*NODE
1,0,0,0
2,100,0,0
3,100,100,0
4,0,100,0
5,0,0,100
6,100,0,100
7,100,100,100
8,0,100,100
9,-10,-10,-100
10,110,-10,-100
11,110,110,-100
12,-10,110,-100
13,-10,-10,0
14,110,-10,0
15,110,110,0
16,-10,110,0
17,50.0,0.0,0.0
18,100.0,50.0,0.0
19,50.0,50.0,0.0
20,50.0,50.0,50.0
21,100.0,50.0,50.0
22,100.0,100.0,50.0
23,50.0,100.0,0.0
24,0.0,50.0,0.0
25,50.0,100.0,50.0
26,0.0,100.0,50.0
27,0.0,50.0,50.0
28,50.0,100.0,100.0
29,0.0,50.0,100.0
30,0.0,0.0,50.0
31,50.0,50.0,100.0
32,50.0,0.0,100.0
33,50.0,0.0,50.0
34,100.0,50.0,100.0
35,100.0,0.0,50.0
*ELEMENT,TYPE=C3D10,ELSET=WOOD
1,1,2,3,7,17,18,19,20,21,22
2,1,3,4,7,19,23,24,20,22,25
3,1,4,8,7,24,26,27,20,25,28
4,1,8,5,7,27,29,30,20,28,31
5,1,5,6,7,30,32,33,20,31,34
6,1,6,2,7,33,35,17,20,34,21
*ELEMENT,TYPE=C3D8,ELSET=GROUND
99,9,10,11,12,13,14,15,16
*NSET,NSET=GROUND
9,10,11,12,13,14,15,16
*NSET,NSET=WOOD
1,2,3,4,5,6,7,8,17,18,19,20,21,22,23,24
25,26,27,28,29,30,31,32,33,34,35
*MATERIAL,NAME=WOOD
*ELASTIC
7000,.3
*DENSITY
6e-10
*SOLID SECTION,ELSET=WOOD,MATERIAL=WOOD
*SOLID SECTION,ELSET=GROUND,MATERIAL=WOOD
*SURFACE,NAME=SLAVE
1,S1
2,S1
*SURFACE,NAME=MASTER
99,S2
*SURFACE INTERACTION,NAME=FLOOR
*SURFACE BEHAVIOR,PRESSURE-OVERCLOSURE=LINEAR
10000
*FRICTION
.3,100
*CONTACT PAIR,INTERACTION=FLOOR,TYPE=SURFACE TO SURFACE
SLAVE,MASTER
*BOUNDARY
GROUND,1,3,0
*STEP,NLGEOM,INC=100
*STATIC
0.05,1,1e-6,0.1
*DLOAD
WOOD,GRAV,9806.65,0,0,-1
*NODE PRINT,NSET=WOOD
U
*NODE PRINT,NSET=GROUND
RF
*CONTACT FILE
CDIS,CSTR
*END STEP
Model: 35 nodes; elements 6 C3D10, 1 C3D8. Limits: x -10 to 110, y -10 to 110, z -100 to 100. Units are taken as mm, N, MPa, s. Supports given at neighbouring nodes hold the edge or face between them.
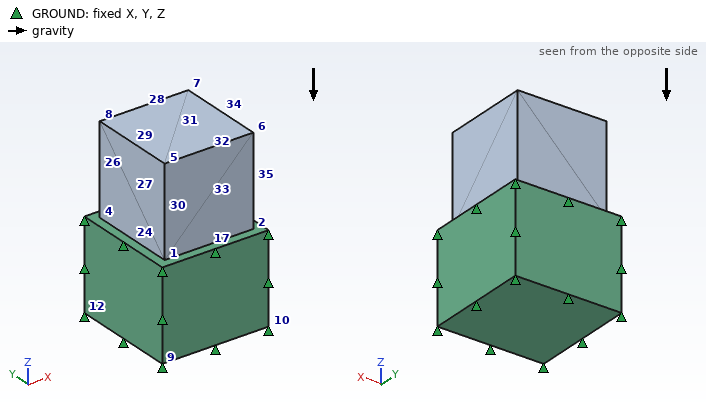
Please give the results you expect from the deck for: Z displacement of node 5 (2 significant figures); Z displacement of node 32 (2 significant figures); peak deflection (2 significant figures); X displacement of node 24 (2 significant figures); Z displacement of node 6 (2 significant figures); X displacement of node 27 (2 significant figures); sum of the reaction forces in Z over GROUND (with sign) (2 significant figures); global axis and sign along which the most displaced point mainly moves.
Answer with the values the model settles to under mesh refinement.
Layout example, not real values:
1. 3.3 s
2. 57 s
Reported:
1. -4.0e-06 mm
2. -4.1e-06 mm
3. 4.3e-06 mm
4. -8.6e-07 mm
5. -3.7e-06 mm
6. -6.7e-07 mm
7. 5.9 N
8. -Z
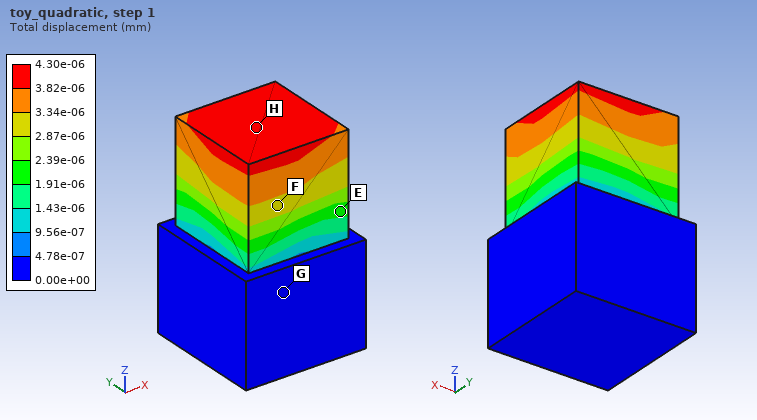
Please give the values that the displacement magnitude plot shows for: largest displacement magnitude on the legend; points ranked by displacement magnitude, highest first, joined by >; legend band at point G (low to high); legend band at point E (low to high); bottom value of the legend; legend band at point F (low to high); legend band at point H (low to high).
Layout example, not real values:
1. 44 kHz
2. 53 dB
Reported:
1. 4.30e-06 mm
2. H > F > E > G
3. 0.00e+00 to 4.78e-07 mm
4. 1.91e-06 to 2.39e-06 mm
5. 0.00e+00 mm
6. 2.87e-06 to 3.34e-06 mm
7. 3.82e-06 to 4.30e-06 mm
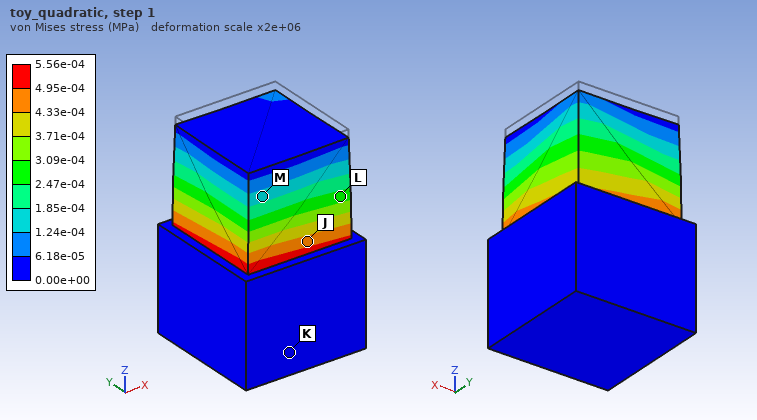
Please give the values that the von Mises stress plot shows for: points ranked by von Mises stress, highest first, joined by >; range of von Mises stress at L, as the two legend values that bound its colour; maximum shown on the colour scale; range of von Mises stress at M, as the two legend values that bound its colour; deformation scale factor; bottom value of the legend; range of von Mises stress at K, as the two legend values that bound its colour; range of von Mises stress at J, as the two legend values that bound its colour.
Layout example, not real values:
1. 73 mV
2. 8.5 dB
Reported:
1. J > L > M > K
2. 2.47e-04 to 3.09e-04 MPa
3. 5.56e-04 MPa
4. 1.24e-04 to 1.85e-04 MPa
5. 2e+06
6. 0.00e+00 MPa
7. 0.00e+00 to 6.18e-05 MPa
8. 4.33e-04 to 4.95e-04 MPa
